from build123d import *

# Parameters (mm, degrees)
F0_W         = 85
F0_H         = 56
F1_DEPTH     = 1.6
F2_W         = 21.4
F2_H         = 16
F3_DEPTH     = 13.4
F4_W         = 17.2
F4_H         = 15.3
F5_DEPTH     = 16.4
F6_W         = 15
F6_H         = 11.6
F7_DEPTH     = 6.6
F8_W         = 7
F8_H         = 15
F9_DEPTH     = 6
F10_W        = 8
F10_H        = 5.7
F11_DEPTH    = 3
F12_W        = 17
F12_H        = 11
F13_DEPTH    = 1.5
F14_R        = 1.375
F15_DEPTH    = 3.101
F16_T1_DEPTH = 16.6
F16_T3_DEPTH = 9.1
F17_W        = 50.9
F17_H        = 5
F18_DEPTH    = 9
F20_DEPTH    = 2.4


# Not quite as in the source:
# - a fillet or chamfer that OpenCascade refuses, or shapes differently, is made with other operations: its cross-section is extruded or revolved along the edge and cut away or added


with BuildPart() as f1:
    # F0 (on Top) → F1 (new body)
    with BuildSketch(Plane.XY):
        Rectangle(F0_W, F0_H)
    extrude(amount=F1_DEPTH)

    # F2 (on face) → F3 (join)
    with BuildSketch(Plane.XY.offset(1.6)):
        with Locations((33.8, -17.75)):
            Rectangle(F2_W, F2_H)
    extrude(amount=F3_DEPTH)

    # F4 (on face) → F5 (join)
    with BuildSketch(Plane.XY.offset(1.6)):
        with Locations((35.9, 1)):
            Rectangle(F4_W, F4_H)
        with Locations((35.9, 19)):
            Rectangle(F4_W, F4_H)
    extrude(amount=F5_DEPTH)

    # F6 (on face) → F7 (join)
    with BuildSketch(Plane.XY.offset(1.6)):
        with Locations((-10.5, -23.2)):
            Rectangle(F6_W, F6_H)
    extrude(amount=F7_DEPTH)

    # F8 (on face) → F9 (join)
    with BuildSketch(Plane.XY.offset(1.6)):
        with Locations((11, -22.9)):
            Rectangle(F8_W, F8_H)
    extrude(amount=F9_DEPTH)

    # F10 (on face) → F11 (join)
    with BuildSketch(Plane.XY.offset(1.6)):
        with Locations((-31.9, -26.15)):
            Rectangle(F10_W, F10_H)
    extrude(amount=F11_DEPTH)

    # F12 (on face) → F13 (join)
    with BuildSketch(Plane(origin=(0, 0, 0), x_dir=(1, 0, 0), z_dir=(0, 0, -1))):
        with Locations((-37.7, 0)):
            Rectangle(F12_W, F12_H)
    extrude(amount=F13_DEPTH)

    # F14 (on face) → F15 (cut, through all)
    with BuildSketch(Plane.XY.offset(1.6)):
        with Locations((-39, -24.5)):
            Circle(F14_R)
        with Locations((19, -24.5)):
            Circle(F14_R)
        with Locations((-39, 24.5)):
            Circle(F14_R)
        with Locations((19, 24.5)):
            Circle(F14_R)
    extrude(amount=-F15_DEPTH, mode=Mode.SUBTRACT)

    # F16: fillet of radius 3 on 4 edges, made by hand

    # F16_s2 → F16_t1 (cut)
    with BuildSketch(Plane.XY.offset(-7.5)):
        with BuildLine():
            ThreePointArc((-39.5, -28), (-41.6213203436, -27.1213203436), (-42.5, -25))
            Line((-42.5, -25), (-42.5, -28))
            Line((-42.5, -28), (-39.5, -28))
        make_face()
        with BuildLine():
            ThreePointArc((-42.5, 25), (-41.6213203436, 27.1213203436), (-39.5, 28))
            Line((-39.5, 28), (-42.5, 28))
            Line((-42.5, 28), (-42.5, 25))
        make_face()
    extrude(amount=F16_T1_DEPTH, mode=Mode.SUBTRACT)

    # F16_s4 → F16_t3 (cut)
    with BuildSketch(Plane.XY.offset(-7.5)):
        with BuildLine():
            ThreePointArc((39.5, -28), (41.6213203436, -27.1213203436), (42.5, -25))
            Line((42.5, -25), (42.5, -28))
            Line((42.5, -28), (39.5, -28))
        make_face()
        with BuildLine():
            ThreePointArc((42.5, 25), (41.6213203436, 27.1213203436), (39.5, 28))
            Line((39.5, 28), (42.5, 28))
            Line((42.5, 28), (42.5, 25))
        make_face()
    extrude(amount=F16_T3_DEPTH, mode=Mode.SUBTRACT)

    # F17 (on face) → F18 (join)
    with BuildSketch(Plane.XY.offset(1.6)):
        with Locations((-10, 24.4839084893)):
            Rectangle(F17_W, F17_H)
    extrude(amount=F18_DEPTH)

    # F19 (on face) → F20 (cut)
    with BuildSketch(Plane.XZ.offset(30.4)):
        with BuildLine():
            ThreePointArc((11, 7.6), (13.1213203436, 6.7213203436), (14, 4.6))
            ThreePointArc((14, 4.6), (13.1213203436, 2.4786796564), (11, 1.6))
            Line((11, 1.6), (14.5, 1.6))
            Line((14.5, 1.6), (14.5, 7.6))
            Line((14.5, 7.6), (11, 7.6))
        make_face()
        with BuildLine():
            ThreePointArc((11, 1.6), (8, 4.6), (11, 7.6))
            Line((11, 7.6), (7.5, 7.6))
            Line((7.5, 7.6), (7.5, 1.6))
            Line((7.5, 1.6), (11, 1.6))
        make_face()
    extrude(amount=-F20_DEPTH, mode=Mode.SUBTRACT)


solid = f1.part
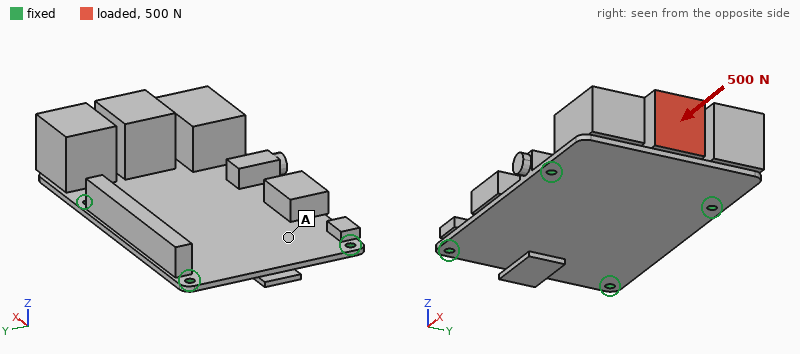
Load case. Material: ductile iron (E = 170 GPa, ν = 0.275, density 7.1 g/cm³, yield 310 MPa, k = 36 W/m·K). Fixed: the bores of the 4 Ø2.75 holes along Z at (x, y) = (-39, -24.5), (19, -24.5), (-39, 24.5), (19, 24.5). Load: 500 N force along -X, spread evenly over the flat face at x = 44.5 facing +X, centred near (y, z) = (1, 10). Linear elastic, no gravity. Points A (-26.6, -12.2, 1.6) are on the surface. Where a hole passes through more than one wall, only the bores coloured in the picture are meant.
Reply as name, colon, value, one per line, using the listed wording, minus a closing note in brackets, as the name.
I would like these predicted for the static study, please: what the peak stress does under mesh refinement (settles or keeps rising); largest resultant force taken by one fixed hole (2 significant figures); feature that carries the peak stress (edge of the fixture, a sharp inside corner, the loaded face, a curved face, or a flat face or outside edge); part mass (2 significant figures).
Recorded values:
what the peak stress does under mesh refinement: keeps rising
largest resultant force taken by one fixed hole: 180 N
feature that carries the peak stress: edge of the fixture
part mass: 180 g
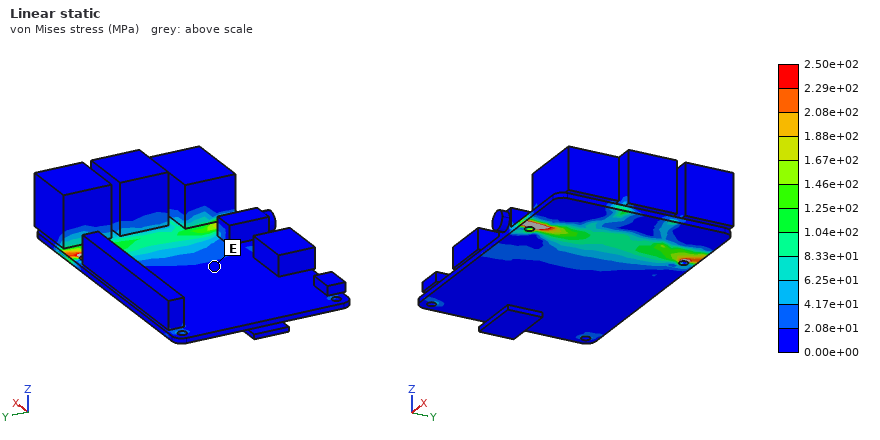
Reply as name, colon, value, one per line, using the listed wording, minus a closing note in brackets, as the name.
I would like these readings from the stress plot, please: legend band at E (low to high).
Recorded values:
legend band at E: 0.00e+00 to 2.08e+01 MPa
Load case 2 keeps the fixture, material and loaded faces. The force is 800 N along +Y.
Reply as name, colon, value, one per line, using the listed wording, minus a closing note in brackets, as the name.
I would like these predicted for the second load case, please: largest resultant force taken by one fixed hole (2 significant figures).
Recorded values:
largest resultant force taken by one fixed hole: 590 N
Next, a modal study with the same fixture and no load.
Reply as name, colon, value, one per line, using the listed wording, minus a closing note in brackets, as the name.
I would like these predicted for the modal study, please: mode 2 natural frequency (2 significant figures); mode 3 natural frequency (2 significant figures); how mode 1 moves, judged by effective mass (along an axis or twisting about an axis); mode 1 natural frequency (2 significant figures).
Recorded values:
mode 2 natural frequency: 1700 Hz
mode 3 natural frequency: 2000 Hz
how mode 1 moves, judged by effective mass: along Z
mode 1 natural frequency: 530 Hz
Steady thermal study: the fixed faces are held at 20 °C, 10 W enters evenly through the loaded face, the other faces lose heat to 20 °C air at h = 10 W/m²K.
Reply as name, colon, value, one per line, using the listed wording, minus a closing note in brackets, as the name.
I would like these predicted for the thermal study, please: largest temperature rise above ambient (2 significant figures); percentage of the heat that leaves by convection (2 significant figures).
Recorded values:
largest temperature rise above ambient: 72 K
percentage of the heat that leaves by convection: 30 %
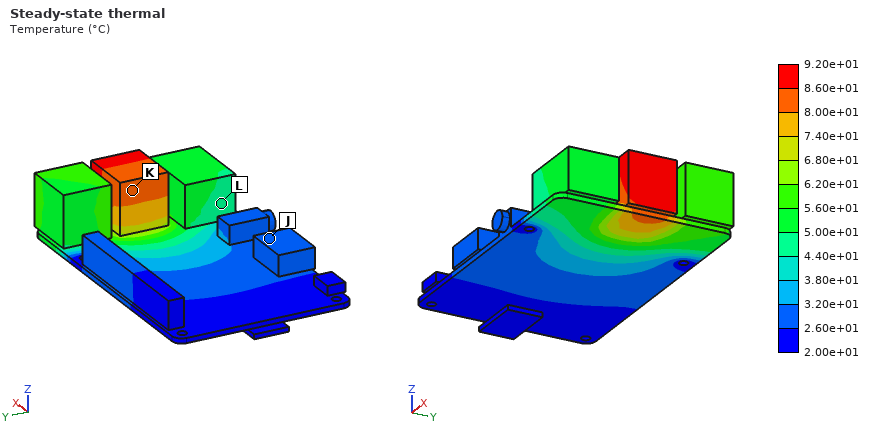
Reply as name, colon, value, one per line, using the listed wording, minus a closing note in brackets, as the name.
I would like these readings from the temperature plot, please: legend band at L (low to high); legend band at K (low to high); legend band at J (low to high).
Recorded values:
legend band at L: 4.40e+01 to 5.00e+01 °C
legend band at K: 8.00e+01 to 8.60e+01 °C
legend band at J: 2.60e+01 to 3.20e+01 °C
